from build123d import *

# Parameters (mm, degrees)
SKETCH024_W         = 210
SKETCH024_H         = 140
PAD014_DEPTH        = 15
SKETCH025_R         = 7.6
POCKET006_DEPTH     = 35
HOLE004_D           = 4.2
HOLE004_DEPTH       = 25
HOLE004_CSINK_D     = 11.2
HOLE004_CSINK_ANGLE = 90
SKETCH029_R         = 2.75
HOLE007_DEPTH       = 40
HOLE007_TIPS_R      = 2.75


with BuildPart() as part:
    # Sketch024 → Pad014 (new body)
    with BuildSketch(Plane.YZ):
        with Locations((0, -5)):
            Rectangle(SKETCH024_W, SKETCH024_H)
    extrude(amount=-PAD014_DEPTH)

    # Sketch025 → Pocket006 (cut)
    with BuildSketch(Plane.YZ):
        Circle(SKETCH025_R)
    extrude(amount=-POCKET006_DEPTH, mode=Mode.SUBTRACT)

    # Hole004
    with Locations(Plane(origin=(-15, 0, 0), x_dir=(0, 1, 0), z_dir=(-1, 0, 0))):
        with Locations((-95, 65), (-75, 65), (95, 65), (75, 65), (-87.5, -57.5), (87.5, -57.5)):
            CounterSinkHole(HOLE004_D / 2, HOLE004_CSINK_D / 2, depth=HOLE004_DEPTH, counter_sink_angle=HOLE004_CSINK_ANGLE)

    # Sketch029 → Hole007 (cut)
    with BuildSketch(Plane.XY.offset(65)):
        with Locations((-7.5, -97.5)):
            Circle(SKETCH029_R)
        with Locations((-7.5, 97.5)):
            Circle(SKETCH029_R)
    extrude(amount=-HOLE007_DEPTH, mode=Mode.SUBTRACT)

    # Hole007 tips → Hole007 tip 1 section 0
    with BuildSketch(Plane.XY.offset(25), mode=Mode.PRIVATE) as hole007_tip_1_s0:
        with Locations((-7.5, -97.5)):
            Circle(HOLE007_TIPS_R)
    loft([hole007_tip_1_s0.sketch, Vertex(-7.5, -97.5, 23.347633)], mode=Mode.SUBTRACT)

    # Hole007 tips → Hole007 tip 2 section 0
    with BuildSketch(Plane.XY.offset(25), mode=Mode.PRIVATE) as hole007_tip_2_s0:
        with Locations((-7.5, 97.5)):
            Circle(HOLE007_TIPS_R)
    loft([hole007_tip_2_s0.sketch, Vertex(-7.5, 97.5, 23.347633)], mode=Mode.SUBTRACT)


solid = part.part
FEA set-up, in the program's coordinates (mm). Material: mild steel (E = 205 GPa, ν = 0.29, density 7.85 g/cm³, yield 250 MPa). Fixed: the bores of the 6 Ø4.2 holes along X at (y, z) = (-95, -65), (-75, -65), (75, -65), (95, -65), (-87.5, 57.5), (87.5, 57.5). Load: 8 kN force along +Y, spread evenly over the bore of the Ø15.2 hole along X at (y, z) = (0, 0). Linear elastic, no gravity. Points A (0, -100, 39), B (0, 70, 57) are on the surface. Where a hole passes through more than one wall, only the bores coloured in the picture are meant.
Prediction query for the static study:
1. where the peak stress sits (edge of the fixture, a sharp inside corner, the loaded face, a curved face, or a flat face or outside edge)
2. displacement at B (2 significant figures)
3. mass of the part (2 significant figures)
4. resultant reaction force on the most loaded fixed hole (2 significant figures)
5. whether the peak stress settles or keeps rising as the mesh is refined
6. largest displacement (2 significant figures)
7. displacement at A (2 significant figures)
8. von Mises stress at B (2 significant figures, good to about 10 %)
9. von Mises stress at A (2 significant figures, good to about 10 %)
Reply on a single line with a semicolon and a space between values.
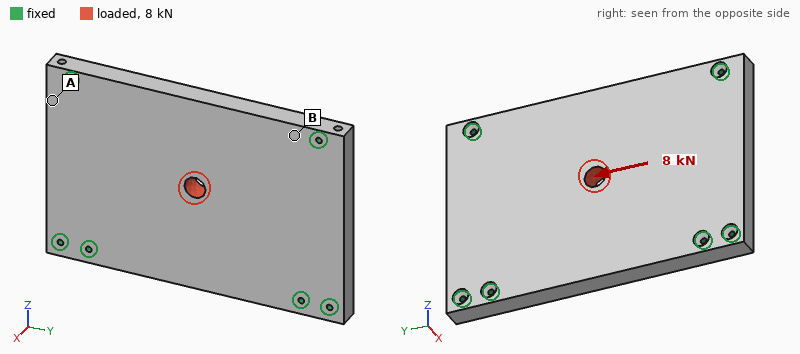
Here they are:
edge of the fixture; 0.55 µm; 3.4 kg; 1.9 kN; keeps rising; 2.6 µm; 0.83 µm; 5.3 MPa; 1.6 MPa
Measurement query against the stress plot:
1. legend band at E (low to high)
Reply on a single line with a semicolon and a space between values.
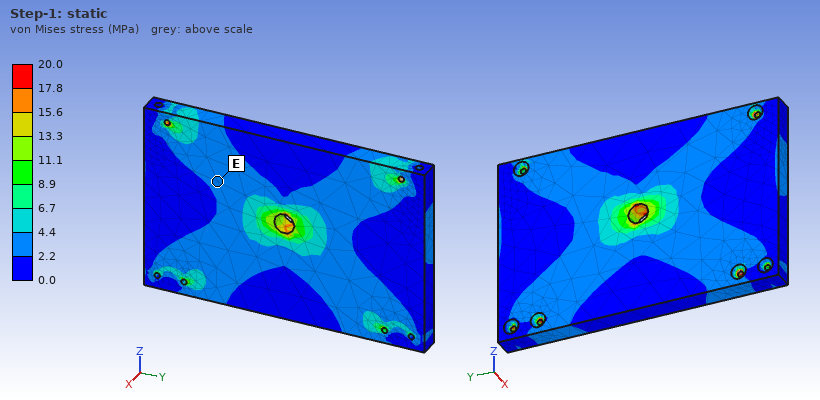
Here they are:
2.2 to 4.4 MPa
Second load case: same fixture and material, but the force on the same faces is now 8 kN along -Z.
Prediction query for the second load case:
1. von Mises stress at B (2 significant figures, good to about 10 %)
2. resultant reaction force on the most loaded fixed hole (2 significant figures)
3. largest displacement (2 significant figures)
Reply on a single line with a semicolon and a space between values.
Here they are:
3.7 MPa; 2.0 kN; 3.6 µm
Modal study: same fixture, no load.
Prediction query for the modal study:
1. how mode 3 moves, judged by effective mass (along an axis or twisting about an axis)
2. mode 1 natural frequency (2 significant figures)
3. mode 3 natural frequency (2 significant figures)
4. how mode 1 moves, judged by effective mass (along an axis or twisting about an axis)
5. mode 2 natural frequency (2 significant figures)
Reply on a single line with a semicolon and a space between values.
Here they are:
twisting about Z; 1800 Hz; 3800 Hz; along X; 3200 Hz
